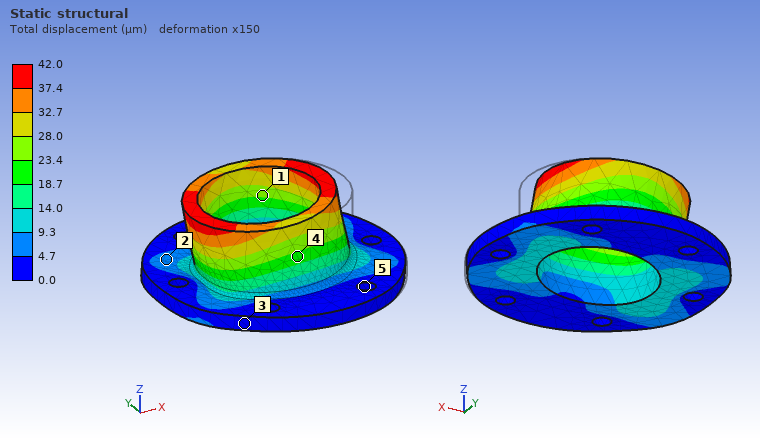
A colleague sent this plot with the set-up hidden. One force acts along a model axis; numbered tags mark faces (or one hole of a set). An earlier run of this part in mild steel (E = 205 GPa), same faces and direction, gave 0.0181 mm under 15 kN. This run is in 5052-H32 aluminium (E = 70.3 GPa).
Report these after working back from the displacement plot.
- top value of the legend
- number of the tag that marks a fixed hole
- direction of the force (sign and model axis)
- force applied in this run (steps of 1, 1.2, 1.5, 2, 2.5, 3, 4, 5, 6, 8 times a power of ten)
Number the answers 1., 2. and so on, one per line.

1. 42.0 µm
2. 5
3. -X
4. 12 kN
